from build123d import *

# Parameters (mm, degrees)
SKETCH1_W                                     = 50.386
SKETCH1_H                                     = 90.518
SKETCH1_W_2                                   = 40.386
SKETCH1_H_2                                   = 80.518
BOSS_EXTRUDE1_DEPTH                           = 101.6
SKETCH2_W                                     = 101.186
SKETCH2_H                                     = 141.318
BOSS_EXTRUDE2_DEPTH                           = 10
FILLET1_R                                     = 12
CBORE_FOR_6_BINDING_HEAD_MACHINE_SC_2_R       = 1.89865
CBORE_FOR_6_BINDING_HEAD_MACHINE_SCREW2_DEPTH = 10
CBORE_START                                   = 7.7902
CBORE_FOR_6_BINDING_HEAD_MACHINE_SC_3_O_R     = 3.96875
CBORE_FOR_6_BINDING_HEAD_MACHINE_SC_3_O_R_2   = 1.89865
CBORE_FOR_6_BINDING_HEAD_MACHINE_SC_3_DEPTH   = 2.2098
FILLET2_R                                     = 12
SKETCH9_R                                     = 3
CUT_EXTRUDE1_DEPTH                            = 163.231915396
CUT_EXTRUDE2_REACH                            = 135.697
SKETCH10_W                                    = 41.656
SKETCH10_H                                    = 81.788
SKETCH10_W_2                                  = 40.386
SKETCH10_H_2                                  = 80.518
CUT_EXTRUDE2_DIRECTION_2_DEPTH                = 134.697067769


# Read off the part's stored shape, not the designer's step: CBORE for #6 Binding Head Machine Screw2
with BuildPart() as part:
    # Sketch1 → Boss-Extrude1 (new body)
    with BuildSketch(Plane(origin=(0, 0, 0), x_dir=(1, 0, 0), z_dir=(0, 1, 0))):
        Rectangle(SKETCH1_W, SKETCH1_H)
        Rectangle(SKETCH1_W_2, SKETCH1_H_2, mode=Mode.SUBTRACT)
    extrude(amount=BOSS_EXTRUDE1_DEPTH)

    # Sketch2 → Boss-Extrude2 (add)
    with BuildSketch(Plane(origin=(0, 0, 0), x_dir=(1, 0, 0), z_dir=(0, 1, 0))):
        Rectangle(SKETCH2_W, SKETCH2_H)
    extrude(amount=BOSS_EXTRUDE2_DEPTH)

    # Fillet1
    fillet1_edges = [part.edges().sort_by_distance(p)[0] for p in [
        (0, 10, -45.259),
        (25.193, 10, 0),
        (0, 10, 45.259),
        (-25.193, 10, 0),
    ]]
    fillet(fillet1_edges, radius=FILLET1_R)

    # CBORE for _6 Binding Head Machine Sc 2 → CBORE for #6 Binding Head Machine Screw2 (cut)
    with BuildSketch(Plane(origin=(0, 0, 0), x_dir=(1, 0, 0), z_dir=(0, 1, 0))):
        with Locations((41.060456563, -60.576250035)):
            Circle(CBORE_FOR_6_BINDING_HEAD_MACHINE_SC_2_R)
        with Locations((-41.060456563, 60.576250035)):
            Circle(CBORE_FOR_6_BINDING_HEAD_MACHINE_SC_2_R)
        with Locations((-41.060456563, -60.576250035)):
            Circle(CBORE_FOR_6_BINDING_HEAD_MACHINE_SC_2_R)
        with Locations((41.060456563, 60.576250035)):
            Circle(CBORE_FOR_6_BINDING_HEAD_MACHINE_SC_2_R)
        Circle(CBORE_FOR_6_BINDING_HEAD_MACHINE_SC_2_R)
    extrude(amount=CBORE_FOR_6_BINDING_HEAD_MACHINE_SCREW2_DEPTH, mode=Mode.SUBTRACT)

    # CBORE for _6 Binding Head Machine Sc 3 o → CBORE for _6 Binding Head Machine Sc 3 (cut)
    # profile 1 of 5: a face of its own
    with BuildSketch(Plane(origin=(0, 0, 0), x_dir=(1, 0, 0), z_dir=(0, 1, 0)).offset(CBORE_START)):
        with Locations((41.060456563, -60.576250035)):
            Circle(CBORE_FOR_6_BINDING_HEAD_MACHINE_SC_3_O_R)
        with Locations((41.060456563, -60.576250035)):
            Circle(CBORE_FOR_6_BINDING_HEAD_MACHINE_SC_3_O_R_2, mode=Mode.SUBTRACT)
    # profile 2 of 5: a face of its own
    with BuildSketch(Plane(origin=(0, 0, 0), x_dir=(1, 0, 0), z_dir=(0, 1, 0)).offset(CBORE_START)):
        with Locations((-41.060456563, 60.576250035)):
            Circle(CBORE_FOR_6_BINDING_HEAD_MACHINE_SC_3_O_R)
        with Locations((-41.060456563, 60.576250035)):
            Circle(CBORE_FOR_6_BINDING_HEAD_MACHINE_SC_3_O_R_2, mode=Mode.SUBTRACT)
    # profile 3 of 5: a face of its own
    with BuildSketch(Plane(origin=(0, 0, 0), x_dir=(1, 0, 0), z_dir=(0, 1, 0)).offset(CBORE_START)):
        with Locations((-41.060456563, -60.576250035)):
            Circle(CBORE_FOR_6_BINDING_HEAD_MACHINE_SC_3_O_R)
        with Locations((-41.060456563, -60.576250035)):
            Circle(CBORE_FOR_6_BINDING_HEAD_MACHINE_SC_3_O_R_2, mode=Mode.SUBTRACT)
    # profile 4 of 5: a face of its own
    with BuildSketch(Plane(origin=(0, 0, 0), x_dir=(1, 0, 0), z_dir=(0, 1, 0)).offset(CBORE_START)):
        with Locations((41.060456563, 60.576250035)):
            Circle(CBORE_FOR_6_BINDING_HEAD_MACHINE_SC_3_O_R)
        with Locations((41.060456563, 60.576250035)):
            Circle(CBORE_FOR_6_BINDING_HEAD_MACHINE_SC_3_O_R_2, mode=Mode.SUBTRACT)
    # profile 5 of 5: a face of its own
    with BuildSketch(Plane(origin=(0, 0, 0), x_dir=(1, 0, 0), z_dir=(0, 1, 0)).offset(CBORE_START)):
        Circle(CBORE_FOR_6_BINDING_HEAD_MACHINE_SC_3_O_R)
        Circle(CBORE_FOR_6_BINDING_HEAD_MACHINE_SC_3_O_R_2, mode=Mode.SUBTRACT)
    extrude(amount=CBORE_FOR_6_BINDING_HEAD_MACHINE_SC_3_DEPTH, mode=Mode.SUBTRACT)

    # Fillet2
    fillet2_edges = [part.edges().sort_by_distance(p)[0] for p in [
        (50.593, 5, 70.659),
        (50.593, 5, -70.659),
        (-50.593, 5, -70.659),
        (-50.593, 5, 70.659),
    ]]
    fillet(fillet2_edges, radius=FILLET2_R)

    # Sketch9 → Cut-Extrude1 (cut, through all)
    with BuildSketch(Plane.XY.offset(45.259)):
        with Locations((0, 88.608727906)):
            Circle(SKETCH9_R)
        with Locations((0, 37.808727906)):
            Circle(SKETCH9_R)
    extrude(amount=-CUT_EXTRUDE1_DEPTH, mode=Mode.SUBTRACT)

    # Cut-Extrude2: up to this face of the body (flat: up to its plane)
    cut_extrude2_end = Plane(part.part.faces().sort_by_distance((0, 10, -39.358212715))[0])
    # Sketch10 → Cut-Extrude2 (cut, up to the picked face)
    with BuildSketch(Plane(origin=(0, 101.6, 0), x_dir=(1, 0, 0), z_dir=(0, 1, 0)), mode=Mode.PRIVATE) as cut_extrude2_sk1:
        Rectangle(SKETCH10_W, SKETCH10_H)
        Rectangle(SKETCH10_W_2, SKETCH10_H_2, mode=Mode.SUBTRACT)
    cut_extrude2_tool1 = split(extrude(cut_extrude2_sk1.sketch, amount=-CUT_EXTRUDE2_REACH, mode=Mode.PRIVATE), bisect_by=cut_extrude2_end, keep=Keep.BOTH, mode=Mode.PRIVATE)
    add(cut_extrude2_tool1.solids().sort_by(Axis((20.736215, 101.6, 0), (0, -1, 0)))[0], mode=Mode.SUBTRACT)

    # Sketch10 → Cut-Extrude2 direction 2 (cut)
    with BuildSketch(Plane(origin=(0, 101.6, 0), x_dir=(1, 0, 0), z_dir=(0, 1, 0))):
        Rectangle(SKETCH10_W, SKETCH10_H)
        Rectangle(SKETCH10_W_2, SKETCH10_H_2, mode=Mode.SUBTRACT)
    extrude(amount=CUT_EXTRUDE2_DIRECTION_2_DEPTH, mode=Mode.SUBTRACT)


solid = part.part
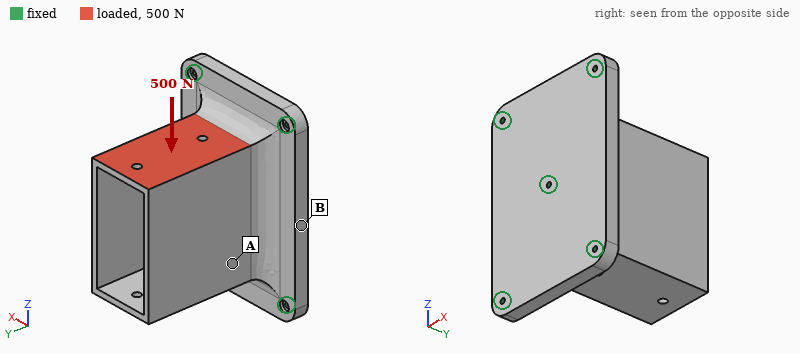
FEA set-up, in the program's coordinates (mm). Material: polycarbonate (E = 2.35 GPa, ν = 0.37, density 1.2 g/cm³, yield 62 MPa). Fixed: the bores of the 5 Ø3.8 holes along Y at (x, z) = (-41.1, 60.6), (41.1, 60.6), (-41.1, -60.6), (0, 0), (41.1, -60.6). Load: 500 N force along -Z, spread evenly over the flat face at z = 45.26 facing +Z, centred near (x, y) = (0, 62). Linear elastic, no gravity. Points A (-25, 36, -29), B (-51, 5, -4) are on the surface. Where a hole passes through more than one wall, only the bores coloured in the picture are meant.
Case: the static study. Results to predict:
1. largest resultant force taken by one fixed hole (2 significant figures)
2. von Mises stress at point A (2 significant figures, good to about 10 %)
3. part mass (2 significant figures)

180 N
1.5 MPa
310 g
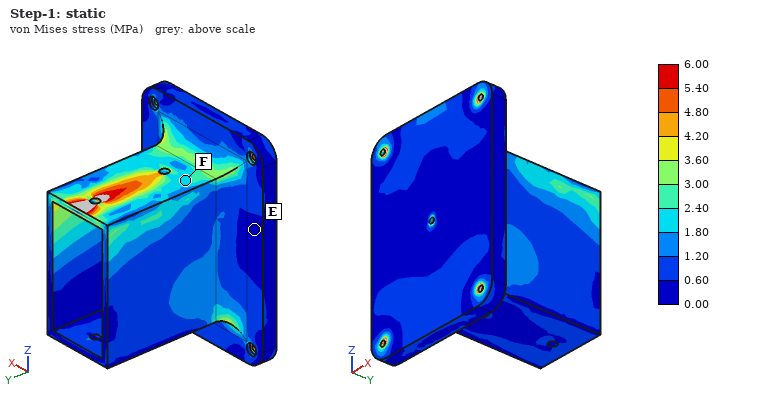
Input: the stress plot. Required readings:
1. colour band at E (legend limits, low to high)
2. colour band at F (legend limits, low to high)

0.00 to 0.60 MPa
1.80 to 2.40 MPa
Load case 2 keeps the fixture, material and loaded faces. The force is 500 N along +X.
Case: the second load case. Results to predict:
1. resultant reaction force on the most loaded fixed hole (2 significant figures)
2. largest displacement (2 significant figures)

370 N
0.62 mm
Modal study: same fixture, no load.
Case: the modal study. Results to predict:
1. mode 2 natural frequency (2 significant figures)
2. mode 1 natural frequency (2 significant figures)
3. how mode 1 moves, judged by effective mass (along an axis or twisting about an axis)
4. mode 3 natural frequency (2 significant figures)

640 Hz
540 Hz
along X
850 Hz
